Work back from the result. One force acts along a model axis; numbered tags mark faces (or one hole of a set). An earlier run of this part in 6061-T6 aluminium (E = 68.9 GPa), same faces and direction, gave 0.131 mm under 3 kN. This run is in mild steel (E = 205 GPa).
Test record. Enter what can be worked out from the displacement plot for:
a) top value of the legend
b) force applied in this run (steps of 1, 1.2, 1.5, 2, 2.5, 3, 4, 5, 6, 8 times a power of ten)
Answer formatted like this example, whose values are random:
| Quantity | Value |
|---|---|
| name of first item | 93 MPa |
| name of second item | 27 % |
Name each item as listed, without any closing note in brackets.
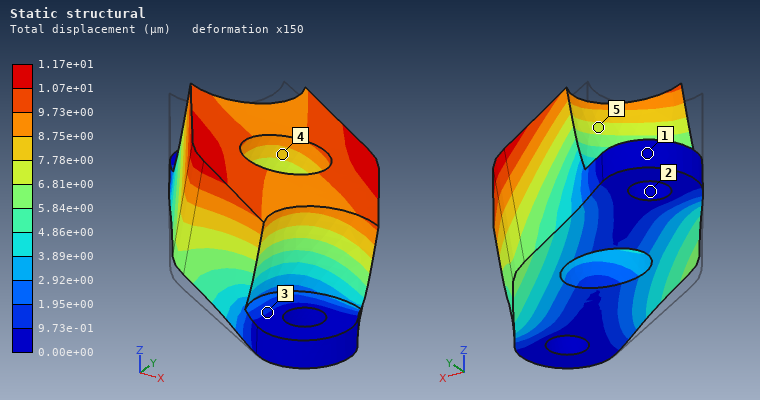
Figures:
| Quantity | Value |
|---|---|
| top value of the legend | 1.17e+01 µm |
| force applied in this run | 800 N |
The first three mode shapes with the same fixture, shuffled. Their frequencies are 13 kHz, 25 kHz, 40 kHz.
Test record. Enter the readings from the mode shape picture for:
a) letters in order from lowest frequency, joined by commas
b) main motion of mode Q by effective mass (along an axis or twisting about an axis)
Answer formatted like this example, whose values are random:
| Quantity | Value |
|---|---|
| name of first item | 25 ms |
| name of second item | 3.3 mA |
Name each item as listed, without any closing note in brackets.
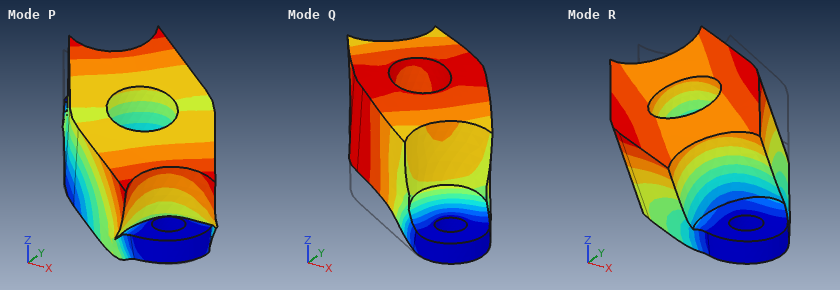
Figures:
| Quantity | Value |
|---|---|
| letters in order from lowest frequency, joined by commas | R, Q, P |
| main motion of mode Q by effective mass | along Z |
